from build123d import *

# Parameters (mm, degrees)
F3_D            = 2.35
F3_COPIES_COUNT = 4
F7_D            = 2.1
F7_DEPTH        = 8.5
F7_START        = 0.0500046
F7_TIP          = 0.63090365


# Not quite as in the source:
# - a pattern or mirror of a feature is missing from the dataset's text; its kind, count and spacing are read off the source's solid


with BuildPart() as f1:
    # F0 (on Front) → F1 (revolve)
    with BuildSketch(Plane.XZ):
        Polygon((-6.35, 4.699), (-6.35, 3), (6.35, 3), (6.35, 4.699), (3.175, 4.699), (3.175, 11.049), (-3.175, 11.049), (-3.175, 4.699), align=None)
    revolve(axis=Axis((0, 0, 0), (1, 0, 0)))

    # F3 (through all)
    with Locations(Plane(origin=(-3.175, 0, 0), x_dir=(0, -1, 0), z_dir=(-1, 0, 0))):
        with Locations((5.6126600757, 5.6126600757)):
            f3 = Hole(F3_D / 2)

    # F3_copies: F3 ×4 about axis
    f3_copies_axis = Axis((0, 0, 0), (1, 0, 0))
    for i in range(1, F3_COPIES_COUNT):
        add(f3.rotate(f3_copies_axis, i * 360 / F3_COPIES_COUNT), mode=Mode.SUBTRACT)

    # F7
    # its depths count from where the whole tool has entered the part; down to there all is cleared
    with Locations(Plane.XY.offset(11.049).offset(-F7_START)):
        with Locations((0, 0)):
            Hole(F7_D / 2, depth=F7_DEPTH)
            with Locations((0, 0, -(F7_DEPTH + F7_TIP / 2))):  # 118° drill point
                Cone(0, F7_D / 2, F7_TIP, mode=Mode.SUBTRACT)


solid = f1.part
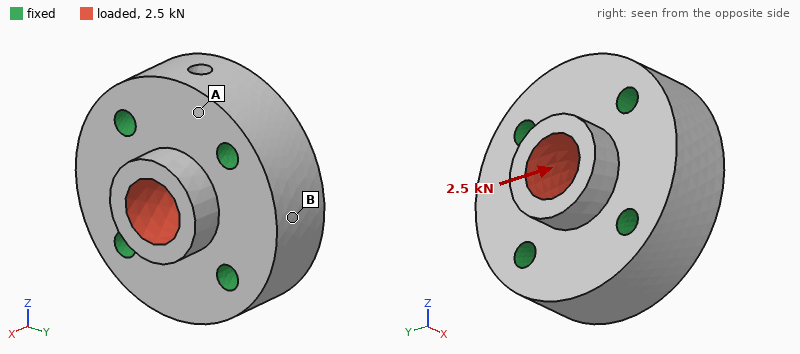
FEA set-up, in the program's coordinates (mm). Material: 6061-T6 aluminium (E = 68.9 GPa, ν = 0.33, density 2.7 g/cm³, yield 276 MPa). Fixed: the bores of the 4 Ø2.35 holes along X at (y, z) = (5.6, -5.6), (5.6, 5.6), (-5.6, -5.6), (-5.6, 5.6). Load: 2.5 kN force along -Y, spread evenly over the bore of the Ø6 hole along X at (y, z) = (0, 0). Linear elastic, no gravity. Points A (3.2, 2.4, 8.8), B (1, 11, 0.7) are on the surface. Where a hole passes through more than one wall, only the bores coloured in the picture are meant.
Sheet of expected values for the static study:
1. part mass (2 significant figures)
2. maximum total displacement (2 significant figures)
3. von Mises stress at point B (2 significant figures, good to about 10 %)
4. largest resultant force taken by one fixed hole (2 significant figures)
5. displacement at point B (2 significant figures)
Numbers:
6.4 g
5.0 µm
9.6 MPa
660 N
0.96 µm
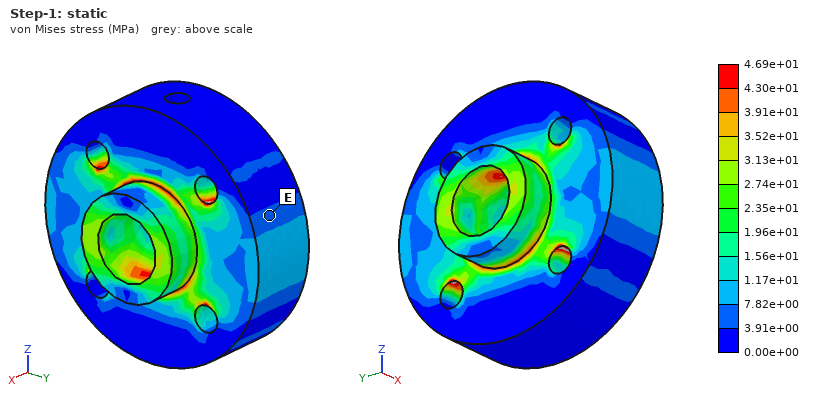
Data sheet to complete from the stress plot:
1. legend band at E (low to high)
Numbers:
3.91e+00 to 7.82e+00 MPa
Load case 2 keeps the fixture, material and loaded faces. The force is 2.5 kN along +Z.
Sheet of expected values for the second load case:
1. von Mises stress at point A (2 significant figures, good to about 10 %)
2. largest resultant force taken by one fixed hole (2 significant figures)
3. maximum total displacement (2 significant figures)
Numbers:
8.8 MPa
660 N
5.1 µm
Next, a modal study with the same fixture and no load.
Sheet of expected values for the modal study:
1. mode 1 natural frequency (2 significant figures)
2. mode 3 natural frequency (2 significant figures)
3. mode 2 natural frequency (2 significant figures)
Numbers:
93 kHz
95 kHz
94 kHz
